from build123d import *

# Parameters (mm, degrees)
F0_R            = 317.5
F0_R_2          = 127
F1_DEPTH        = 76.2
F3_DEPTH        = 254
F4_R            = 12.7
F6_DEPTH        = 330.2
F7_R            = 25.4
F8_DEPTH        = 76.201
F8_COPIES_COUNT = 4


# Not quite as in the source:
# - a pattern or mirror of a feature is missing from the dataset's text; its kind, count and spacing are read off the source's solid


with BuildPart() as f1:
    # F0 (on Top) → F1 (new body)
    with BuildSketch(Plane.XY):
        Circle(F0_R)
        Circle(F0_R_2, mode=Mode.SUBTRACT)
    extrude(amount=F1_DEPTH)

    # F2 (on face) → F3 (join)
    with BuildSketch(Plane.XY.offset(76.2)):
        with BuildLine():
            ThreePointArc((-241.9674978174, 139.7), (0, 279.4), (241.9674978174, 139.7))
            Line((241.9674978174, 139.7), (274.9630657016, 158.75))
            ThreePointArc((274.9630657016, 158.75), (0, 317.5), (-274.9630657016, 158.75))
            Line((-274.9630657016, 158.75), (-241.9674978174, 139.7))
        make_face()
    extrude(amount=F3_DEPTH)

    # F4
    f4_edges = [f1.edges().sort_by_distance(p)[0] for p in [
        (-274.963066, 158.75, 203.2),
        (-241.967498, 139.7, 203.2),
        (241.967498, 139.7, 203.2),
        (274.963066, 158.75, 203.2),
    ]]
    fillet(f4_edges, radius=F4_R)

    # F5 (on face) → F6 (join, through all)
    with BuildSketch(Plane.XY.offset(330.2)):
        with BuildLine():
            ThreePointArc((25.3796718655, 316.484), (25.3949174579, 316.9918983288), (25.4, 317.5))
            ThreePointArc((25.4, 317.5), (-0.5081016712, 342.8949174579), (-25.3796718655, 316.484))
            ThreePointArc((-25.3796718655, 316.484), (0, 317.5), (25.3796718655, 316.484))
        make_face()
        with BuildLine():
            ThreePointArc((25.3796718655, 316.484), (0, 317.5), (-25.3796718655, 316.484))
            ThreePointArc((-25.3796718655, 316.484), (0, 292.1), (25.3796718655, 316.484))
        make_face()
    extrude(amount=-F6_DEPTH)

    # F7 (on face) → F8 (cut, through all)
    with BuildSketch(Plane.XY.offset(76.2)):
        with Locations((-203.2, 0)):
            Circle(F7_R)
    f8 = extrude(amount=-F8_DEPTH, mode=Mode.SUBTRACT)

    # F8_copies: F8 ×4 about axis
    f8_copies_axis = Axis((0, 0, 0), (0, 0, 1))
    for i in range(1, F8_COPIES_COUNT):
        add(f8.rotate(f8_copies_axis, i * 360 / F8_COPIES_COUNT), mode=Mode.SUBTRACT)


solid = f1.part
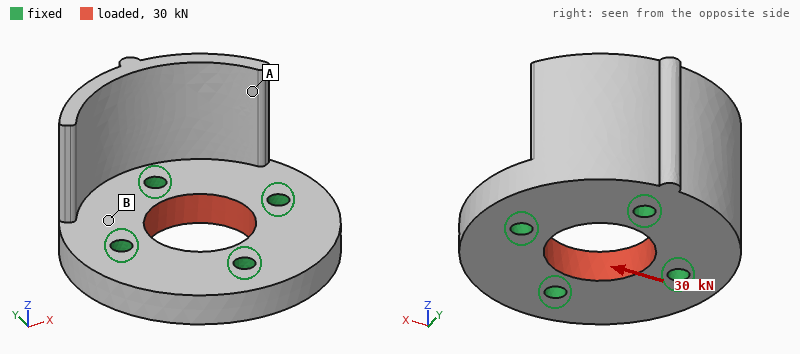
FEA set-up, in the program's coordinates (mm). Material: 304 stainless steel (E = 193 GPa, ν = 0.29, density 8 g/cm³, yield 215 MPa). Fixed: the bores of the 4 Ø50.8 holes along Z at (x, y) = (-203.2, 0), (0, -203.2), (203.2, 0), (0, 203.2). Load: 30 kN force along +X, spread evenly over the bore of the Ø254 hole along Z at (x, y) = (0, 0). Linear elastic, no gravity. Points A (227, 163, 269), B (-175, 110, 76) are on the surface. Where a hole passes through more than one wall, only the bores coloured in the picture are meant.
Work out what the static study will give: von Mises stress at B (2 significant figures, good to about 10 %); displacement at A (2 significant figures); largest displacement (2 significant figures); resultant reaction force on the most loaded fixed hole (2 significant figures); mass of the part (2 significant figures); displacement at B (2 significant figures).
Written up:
0.31 MPa
0.28 µm
0.50 µm
7.6 kN
210 kg
0.30 µm
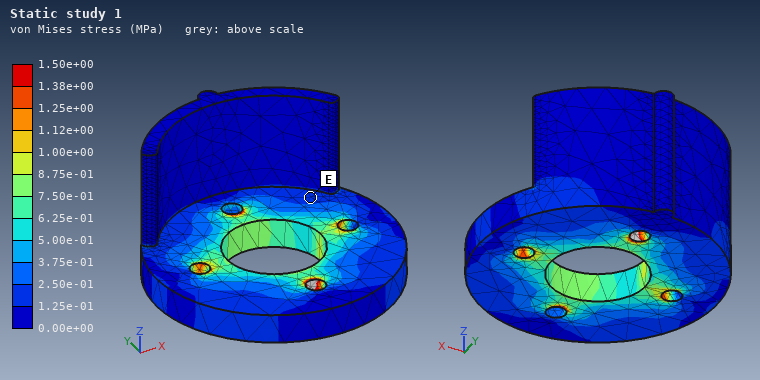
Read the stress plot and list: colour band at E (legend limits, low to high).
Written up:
1.25e-01 to 2.50e-01 MPa
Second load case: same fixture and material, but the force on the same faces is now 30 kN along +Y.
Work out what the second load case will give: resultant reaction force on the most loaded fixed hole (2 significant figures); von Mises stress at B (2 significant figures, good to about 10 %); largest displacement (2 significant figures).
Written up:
7.6 kN
0.29 MPa
0.49 µm
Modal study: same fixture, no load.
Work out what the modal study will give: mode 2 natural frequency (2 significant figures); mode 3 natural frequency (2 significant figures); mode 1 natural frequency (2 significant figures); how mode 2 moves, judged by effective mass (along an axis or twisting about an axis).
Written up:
670 Hz
890 Hz
520 Hz
along Y
